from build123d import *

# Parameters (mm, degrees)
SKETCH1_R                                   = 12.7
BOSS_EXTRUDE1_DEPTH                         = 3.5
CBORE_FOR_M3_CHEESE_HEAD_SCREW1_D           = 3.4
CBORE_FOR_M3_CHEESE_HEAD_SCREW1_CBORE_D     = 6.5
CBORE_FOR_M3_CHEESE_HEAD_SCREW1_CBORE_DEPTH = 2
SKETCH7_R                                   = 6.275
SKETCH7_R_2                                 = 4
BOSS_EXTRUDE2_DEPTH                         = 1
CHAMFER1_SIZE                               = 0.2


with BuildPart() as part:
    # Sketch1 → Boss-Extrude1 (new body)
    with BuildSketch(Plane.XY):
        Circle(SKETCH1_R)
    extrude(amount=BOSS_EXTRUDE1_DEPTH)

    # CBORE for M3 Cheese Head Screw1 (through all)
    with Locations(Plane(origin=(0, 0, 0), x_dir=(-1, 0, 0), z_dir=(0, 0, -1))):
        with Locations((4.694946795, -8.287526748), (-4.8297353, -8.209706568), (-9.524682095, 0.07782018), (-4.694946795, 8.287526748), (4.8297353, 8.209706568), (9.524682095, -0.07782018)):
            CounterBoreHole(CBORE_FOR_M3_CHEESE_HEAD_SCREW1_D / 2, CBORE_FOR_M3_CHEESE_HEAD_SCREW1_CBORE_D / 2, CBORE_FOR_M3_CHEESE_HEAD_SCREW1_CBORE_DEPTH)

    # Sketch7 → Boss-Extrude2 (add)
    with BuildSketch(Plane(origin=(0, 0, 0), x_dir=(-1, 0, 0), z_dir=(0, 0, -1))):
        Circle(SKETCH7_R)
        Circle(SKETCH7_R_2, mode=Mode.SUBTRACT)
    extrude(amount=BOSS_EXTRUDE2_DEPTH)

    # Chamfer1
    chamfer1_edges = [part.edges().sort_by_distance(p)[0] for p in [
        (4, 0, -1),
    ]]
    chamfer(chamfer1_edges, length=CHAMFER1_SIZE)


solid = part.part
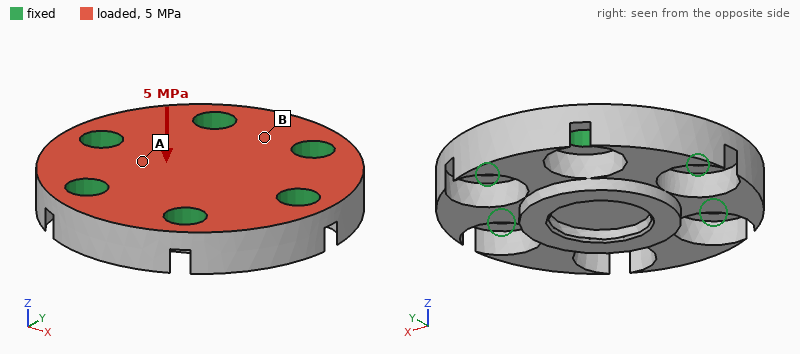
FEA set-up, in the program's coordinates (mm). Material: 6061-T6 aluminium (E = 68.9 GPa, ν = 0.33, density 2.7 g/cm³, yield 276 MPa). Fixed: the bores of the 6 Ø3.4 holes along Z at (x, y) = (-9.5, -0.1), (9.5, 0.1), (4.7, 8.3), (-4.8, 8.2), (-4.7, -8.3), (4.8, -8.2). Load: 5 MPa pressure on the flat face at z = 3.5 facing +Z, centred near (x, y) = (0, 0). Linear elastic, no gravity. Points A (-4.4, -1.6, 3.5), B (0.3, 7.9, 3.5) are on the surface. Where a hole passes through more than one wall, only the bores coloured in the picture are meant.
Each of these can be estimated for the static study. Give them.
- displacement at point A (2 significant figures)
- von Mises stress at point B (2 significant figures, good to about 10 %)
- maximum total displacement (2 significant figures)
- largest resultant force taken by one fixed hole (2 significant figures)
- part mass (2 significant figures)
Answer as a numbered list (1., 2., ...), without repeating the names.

1. 3.5 µm
2. 18 MPa
3. 4.5 µm
4. 380 N
5. 3.7 g
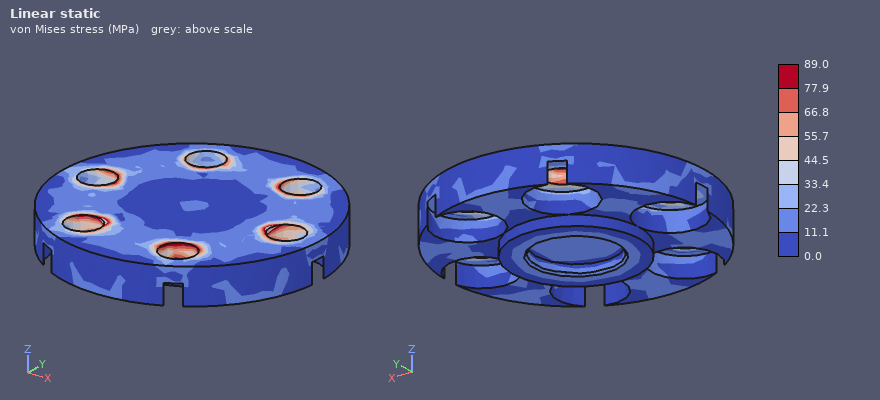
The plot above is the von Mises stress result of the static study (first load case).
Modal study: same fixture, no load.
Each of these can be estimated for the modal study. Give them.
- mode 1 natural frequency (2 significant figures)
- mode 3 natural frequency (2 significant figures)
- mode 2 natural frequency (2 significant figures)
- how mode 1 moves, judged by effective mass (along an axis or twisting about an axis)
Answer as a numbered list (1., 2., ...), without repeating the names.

1. 60 kHz
2. 77 kHz
3. 77 kHz
4. along Z
